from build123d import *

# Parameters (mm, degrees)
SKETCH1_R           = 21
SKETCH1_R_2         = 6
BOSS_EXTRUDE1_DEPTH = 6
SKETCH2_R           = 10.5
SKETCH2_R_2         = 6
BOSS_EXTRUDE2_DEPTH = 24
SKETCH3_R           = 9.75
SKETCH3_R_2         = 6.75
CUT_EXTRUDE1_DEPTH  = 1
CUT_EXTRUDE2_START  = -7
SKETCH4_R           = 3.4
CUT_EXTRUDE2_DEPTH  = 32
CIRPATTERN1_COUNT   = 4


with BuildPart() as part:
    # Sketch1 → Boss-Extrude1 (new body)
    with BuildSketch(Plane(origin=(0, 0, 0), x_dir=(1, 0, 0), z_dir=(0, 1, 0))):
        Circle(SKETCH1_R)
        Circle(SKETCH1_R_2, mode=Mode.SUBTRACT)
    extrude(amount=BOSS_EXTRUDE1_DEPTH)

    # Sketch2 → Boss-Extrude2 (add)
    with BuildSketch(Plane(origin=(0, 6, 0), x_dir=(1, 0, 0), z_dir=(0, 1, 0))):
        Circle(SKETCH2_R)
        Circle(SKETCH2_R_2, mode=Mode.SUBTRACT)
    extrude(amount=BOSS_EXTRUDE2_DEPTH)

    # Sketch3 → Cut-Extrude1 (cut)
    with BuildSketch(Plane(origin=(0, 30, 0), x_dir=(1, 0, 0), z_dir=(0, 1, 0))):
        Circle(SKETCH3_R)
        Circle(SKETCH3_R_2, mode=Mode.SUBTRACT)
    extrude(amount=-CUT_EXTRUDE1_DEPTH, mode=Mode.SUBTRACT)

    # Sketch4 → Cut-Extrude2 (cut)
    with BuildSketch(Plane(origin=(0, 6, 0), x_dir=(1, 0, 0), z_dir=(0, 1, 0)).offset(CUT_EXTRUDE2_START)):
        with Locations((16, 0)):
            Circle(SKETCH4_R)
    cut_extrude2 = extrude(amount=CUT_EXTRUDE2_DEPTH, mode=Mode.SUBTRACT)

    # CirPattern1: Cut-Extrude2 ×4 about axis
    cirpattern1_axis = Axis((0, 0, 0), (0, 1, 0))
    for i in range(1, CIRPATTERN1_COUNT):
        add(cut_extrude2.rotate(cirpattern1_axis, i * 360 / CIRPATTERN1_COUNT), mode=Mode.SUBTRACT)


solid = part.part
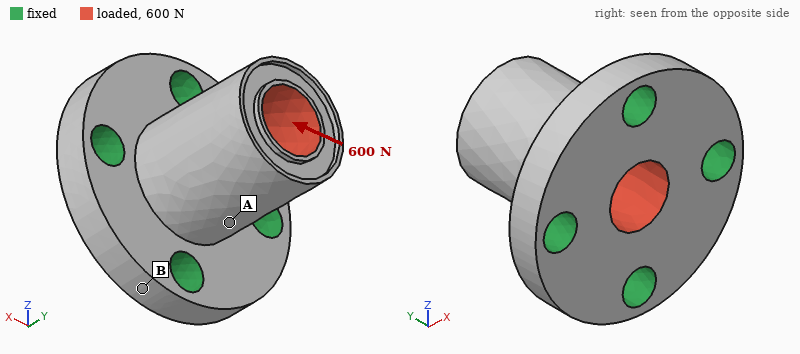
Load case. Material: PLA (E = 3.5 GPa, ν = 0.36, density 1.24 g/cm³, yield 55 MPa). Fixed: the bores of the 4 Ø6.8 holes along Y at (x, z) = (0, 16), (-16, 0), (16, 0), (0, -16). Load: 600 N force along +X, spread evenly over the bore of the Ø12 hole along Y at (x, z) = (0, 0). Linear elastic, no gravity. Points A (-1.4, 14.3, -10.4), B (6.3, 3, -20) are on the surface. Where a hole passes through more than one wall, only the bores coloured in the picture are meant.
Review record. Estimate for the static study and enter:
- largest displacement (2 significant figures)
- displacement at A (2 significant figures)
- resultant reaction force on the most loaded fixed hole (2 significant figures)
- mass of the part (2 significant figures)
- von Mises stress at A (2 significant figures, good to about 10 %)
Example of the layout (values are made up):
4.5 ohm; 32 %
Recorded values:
0.11 mm; 0.039 mm; 330 N; 15 g; 3.2 MPa
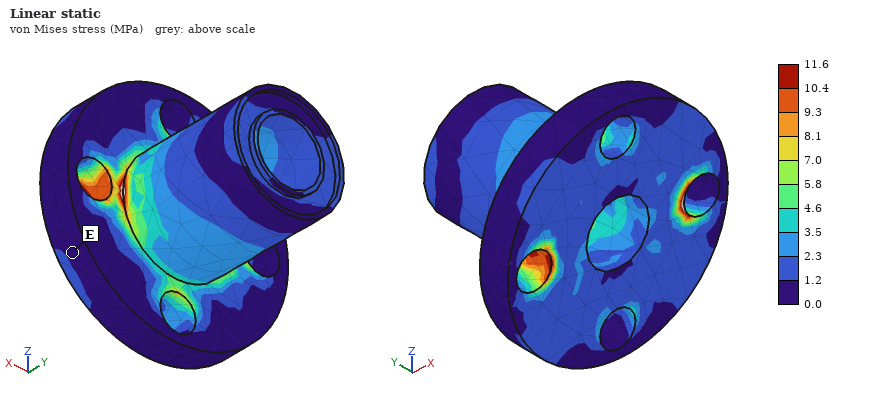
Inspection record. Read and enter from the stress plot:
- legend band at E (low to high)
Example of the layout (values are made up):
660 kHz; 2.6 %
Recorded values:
0.0 to 1.2 MPa
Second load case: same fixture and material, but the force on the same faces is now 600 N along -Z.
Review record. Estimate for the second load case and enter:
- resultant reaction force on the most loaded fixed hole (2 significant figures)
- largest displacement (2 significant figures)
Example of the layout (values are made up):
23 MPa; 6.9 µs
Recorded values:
330 N; 0.11 mm
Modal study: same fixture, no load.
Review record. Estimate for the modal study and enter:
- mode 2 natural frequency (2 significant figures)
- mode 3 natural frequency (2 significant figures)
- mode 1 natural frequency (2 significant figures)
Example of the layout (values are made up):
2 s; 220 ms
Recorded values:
5000 Hz; 9800 Hz; 5000 Hz
